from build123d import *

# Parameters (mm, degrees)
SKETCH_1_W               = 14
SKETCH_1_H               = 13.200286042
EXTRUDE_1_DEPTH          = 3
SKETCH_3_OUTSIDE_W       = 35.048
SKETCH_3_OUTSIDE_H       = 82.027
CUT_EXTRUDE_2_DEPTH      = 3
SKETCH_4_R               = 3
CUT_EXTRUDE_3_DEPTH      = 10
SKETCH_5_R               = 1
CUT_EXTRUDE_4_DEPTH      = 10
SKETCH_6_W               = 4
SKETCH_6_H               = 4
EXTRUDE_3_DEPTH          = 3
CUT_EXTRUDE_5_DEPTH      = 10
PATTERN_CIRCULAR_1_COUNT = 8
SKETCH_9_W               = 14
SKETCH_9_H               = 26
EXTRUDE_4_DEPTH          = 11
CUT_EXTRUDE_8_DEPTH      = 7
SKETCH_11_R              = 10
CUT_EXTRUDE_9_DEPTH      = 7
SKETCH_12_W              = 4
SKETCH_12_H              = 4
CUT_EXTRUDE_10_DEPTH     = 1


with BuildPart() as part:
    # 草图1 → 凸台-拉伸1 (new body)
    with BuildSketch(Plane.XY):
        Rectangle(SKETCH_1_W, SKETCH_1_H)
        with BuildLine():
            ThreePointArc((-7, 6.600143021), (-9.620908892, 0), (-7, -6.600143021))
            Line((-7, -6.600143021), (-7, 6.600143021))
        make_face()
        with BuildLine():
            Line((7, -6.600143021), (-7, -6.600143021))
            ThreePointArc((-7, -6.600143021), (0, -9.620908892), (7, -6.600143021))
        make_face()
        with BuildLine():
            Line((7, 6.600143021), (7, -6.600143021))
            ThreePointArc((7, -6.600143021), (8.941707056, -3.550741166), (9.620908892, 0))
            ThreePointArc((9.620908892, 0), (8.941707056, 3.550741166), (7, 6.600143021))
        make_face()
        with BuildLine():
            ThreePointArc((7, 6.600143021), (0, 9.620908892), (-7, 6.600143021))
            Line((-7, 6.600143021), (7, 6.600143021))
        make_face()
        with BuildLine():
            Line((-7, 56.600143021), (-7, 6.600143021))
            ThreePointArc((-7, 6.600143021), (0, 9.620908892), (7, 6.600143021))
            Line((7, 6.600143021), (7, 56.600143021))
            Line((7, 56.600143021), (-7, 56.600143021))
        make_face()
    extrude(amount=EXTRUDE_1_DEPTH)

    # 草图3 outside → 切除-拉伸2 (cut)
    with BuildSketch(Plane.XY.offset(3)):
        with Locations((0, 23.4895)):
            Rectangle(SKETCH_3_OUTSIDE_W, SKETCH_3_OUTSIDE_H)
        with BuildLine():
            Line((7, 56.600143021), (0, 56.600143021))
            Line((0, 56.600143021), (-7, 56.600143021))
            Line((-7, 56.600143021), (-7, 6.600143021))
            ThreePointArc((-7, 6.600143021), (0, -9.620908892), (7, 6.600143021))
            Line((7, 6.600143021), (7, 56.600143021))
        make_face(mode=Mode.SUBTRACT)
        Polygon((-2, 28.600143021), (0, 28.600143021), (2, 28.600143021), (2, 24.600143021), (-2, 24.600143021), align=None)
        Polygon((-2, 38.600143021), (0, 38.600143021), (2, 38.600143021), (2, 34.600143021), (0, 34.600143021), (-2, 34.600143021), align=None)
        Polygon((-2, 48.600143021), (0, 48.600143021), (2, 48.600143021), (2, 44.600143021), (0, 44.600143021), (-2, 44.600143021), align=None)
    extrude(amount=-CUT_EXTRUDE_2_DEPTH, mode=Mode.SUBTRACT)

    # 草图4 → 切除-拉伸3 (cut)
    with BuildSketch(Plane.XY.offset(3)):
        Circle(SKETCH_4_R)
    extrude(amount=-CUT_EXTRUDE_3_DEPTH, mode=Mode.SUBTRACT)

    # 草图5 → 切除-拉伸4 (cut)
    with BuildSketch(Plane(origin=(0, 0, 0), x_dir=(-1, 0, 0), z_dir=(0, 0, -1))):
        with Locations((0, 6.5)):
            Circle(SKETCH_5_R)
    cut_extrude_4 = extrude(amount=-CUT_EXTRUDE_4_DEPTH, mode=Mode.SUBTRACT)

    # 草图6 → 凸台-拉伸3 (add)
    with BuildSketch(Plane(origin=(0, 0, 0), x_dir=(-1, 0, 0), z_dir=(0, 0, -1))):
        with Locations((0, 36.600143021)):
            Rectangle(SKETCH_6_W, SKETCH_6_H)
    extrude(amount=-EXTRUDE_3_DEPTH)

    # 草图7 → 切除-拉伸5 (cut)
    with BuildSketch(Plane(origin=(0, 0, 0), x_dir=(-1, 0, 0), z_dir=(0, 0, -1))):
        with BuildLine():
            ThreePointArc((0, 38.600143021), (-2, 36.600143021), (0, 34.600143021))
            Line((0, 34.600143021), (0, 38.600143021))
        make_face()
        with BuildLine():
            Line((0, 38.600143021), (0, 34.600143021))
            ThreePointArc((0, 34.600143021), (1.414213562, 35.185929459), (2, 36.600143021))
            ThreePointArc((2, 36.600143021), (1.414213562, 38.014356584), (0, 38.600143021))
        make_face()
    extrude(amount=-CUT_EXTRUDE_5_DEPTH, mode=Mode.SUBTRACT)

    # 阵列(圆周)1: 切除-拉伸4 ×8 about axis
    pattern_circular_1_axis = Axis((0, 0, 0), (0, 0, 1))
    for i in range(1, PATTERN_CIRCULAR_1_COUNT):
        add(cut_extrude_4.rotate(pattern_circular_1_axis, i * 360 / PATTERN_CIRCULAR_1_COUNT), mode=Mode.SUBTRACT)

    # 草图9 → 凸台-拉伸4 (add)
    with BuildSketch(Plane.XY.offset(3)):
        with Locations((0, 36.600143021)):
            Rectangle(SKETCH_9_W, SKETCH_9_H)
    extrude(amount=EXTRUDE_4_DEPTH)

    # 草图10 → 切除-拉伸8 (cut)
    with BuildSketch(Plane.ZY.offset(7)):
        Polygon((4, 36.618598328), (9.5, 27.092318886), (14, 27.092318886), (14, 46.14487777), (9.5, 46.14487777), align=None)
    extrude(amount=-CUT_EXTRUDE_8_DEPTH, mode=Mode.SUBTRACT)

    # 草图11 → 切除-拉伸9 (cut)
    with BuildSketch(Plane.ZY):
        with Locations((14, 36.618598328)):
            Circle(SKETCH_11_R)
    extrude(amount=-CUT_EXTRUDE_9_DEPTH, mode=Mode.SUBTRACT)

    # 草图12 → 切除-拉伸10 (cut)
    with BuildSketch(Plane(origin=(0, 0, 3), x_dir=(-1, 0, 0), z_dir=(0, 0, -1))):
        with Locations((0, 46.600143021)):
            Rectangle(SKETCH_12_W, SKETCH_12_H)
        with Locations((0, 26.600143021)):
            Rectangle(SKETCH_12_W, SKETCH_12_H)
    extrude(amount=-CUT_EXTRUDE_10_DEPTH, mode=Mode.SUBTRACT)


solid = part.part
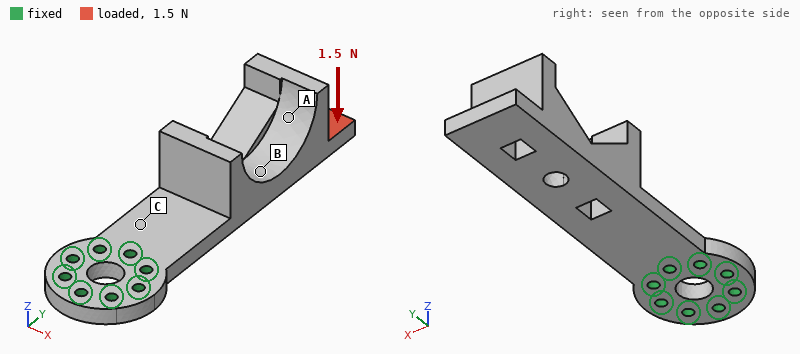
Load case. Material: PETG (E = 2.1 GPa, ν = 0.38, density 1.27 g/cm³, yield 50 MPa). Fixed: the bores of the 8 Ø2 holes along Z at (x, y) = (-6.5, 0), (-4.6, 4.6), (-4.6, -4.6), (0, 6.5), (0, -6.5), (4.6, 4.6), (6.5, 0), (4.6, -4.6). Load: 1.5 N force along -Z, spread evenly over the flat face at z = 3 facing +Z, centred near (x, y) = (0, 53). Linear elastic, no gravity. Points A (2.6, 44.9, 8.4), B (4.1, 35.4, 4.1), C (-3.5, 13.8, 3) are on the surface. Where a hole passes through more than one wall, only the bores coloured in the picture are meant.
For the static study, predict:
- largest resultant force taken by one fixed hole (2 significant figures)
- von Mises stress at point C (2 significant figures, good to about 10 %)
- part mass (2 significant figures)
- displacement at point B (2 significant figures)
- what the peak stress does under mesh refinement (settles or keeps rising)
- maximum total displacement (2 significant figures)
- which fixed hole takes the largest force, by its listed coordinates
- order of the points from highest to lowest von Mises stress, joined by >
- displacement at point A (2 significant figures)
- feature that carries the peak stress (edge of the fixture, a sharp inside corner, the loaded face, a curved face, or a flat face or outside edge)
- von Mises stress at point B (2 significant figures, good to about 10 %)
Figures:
6.9 N
2.7 MPa
5.7 g
0.32 mm
keeps rising
0.68 mm
(0, 6.5)
C > B > A
0.49 mm
edge of the fixture
0.64 MPa
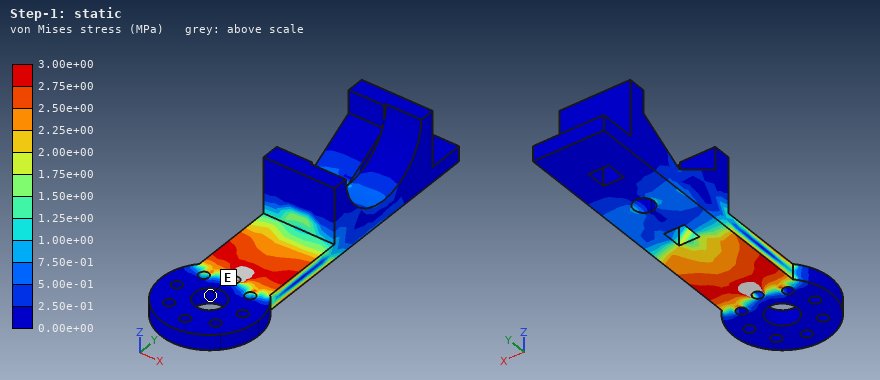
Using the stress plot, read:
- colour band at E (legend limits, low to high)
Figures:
0.00e+00 to 2.50e-01 MPa
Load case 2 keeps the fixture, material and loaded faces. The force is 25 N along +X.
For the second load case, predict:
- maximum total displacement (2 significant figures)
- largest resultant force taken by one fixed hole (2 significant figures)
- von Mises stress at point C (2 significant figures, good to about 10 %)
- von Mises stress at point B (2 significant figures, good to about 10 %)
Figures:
0.72 mm
93 N
5.7 MPa
3.2 MPa
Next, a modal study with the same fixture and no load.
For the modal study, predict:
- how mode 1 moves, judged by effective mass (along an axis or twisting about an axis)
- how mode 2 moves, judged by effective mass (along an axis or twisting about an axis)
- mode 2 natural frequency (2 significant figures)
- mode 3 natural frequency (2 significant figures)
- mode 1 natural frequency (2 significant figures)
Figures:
along Z
along X
690 Hz
1100 Hz
190 Hz
